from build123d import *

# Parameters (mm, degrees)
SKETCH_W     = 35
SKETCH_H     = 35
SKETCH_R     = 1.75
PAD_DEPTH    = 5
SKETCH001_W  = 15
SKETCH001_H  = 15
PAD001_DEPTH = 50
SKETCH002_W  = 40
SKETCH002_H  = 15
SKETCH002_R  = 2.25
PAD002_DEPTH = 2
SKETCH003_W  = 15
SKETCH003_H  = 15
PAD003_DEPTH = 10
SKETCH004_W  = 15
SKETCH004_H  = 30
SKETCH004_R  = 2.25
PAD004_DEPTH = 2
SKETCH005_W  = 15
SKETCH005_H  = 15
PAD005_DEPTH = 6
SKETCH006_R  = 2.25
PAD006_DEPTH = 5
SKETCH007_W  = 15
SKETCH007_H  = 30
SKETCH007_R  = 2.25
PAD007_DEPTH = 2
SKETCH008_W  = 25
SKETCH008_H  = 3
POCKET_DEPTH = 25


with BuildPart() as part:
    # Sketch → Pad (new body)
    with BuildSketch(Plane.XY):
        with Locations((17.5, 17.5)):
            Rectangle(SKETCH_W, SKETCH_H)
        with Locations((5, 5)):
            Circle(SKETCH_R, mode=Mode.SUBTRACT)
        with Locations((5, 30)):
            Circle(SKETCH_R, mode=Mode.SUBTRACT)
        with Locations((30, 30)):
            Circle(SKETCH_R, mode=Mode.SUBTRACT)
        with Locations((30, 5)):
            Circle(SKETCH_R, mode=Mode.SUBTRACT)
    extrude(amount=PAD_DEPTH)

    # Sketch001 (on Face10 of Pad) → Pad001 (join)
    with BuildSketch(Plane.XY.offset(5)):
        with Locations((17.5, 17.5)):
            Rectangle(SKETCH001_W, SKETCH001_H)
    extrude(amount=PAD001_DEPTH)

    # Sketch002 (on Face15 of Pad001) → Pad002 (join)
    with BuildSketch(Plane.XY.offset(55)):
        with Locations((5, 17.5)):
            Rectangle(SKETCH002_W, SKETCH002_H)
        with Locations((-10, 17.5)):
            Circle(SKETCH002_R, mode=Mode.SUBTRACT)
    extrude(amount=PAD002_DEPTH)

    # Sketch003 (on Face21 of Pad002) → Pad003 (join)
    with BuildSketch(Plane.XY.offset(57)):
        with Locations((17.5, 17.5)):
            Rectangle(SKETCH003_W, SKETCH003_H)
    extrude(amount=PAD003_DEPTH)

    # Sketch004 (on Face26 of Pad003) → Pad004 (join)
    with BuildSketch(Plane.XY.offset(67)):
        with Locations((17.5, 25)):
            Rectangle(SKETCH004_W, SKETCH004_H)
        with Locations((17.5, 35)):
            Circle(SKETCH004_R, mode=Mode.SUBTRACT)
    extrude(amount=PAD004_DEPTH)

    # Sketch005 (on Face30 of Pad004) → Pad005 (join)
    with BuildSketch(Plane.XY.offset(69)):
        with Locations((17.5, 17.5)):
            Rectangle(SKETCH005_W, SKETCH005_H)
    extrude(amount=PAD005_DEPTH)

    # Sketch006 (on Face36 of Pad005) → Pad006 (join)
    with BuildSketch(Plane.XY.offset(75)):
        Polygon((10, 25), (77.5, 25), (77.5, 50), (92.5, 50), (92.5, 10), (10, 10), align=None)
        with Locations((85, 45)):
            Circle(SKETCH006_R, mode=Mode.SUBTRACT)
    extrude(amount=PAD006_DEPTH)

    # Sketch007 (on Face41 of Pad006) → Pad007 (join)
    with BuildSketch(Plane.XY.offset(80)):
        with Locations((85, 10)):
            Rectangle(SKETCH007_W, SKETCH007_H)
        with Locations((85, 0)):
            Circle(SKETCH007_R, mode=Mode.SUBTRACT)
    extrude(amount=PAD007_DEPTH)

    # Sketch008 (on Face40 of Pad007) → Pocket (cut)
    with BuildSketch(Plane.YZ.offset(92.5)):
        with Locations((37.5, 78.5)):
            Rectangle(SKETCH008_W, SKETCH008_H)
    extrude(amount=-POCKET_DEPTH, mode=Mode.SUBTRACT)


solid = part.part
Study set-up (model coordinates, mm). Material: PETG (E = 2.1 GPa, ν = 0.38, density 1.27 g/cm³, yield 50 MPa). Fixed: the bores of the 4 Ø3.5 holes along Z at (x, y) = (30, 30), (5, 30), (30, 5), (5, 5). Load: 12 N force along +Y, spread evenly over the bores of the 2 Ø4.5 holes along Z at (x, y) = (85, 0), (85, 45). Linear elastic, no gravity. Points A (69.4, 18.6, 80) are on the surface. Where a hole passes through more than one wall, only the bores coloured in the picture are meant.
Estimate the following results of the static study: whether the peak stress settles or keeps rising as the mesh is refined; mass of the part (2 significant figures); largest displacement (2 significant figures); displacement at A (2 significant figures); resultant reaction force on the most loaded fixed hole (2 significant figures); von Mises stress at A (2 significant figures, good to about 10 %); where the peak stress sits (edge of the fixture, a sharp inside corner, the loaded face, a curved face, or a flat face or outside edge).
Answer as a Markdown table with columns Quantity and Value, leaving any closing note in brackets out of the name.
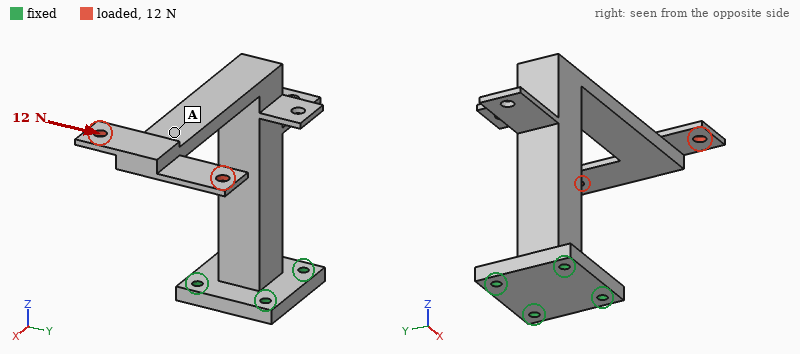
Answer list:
| Quantity | Value |
|---|---|
| whether the peak stress settles or keeps rising as the mesh is refined | keeps rising |
| mass of the part | 39 g |
| largest displacement | 1.6 mm |
| displacement at A | 1.1 mm |
| resultant reaction force on the most loaded fixed hole | 24 N |
| von Mises stress at A | 0.60 MPa |
| where the peak stress sits | a sharp inside corner |
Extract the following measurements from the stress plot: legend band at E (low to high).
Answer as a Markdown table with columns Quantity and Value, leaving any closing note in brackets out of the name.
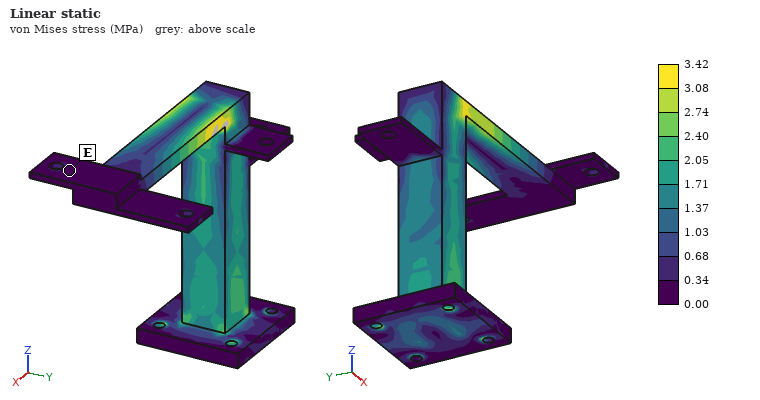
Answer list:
| Quantity | Value |
|---|---|
| legend band at E | 0.00 to 0.34 MPa |
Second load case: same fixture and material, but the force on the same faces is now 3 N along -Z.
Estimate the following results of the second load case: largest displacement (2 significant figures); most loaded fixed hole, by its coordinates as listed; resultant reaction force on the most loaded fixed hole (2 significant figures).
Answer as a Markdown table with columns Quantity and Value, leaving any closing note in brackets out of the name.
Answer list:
| Quantity | Value |
|---|---|
| largest displacement | 1.4 mm |
| most loaded fixed hole, by its coordinates as listed | (30, 30) |
| resultant reaction force on the most loaded fixed hole | 5.7 N |
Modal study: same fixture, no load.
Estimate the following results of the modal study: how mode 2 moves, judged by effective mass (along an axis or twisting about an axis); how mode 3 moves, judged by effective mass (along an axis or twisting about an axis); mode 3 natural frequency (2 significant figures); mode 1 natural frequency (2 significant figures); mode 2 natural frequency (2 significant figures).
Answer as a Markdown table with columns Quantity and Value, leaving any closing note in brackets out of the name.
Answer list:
| Quantity | Value |
|---|---|
| how mode 2 moves, judged by effective mass | along Y |
| how mode 3 moves, judged by effective mass | along X |
| mode 3 natural frequency | 290 Hz |
| mode 1 natural frequency | 140 Hz |
| mode 2 natural frequency | 200 Hz |
